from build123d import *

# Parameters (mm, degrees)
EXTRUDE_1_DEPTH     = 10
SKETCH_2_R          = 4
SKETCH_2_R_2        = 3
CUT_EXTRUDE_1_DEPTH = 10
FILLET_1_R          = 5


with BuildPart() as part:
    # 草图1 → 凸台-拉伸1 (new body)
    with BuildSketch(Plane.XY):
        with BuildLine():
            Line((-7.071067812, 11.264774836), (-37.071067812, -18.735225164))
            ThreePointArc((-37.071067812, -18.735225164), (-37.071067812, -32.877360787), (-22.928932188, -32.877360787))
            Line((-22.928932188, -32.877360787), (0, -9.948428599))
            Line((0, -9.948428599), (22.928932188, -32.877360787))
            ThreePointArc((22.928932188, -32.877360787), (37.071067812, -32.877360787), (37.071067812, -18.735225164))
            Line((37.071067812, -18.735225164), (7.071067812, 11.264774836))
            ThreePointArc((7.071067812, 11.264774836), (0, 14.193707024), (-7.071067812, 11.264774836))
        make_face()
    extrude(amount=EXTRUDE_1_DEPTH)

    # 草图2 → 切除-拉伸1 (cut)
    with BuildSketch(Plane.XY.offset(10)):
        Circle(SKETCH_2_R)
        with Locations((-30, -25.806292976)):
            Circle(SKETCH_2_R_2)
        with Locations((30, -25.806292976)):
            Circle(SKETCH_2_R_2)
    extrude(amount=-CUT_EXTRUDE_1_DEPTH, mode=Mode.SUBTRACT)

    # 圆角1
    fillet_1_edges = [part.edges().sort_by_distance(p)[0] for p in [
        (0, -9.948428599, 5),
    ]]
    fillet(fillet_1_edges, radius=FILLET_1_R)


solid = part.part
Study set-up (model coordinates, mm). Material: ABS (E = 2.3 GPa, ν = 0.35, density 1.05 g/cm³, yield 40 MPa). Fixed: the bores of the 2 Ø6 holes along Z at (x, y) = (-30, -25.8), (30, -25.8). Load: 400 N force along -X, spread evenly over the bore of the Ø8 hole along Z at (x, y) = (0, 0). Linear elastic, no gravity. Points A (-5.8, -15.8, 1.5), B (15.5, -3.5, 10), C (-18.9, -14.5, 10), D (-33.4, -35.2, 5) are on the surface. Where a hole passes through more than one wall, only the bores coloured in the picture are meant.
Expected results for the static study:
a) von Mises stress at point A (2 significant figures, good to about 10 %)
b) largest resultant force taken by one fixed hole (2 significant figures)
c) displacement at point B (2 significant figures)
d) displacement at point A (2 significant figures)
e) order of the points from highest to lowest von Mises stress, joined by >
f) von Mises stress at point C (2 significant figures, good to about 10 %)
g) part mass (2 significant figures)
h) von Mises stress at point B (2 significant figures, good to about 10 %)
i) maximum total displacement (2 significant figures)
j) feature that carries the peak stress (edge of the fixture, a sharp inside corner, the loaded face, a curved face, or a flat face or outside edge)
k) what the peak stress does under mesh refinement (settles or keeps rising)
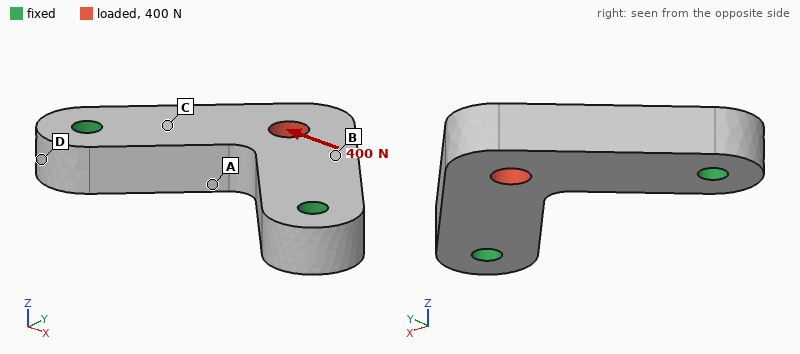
2.0 MPa
250 N
28 µm
19 µm
A > C > B > D
1.4 MPa
20 g
1.1 MPa
43 µm
edge of the fixture
keeps rising
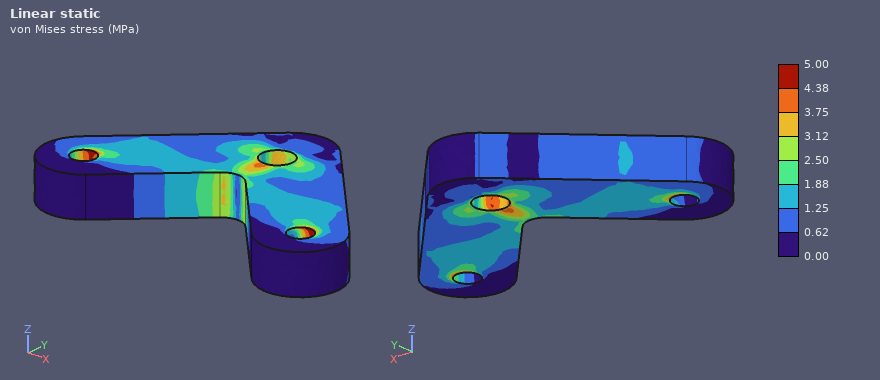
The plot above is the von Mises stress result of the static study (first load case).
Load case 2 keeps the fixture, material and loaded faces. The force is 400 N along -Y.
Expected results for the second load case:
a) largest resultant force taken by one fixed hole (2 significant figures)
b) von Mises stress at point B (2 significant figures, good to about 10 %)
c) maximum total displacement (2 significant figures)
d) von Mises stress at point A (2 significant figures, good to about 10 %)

260 N
1.3 MPa
38 µm
1.2 MPa
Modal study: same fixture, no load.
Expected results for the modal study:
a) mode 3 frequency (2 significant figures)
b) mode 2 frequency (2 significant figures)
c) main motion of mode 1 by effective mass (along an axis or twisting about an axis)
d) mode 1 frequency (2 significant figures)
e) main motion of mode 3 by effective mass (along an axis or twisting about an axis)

5200 Hz
4600 Hz
along Z
1500 Hz
along Z
